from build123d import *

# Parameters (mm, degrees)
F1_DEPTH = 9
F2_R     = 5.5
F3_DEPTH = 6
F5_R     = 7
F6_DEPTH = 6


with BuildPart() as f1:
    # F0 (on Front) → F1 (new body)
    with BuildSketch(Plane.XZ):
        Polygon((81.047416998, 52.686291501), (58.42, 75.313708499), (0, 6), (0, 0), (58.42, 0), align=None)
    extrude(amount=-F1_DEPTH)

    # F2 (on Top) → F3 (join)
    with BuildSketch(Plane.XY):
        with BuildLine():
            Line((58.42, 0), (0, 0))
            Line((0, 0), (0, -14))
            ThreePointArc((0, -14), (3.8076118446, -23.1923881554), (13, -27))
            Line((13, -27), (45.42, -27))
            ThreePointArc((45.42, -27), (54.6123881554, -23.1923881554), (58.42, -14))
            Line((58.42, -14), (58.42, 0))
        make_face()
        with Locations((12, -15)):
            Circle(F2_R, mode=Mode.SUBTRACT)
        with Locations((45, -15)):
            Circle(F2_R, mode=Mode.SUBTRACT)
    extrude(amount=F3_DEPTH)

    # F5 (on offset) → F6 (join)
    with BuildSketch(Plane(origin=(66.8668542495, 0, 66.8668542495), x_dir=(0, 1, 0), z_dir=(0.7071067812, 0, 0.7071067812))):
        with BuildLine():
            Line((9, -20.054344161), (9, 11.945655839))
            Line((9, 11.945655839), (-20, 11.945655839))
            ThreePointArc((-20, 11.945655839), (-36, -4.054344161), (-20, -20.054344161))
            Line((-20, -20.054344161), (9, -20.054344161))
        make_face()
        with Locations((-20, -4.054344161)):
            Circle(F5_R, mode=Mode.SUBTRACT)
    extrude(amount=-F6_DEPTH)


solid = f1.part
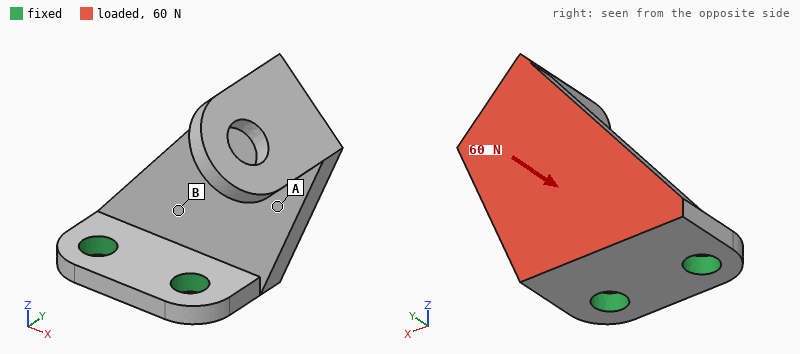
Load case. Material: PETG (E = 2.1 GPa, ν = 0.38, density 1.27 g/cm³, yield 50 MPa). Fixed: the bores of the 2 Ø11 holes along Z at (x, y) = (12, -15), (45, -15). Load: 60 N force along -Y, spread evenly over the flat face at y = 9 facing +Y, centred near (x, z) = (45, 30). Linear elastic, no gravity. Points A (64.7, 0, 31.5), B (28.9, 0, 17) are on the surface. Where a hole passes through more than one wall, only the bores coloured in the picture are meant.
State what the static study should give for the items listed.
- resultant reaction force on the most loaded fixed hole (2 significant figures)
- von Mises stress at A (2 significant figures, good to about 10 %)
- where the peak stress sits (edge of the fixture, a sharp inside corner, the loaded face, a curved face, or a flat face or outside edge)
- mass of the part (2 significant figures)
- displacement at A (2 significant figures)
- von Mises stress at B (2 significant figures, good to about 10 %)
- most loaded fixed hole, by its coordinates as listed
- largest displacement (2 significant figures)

55 N
0.61 MPa
a flat face or outside edge
54 g
0.41 mm
1.7 MPa
(45, -15)
1.1 mm
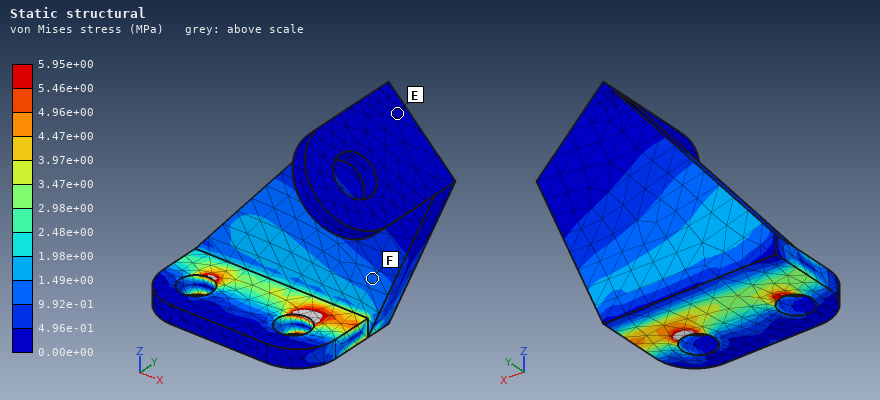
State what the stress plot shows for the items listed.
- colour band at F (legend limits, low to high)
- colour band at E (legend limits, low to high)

9.92e-01 to 1.49e+00 MPa
0.00e+00 to 4.96e-01 MPa
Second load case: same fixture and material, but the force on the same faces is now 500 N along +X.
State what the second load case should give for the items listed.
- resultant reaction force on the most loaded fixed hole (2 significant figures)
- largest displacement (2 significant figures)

510 N
1.0 mm
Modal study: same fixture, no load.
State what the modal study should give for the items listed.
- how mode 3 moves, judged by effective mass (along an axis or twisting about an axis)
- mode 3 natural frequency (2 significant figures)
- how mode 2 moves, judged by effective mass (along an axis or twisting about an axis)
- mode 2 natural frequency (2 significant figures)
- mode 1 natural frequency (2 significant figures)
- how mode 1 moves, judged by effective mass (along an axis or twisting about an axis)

along Z
680 Hz
along X
460 Hz
200 Hz
along Y
